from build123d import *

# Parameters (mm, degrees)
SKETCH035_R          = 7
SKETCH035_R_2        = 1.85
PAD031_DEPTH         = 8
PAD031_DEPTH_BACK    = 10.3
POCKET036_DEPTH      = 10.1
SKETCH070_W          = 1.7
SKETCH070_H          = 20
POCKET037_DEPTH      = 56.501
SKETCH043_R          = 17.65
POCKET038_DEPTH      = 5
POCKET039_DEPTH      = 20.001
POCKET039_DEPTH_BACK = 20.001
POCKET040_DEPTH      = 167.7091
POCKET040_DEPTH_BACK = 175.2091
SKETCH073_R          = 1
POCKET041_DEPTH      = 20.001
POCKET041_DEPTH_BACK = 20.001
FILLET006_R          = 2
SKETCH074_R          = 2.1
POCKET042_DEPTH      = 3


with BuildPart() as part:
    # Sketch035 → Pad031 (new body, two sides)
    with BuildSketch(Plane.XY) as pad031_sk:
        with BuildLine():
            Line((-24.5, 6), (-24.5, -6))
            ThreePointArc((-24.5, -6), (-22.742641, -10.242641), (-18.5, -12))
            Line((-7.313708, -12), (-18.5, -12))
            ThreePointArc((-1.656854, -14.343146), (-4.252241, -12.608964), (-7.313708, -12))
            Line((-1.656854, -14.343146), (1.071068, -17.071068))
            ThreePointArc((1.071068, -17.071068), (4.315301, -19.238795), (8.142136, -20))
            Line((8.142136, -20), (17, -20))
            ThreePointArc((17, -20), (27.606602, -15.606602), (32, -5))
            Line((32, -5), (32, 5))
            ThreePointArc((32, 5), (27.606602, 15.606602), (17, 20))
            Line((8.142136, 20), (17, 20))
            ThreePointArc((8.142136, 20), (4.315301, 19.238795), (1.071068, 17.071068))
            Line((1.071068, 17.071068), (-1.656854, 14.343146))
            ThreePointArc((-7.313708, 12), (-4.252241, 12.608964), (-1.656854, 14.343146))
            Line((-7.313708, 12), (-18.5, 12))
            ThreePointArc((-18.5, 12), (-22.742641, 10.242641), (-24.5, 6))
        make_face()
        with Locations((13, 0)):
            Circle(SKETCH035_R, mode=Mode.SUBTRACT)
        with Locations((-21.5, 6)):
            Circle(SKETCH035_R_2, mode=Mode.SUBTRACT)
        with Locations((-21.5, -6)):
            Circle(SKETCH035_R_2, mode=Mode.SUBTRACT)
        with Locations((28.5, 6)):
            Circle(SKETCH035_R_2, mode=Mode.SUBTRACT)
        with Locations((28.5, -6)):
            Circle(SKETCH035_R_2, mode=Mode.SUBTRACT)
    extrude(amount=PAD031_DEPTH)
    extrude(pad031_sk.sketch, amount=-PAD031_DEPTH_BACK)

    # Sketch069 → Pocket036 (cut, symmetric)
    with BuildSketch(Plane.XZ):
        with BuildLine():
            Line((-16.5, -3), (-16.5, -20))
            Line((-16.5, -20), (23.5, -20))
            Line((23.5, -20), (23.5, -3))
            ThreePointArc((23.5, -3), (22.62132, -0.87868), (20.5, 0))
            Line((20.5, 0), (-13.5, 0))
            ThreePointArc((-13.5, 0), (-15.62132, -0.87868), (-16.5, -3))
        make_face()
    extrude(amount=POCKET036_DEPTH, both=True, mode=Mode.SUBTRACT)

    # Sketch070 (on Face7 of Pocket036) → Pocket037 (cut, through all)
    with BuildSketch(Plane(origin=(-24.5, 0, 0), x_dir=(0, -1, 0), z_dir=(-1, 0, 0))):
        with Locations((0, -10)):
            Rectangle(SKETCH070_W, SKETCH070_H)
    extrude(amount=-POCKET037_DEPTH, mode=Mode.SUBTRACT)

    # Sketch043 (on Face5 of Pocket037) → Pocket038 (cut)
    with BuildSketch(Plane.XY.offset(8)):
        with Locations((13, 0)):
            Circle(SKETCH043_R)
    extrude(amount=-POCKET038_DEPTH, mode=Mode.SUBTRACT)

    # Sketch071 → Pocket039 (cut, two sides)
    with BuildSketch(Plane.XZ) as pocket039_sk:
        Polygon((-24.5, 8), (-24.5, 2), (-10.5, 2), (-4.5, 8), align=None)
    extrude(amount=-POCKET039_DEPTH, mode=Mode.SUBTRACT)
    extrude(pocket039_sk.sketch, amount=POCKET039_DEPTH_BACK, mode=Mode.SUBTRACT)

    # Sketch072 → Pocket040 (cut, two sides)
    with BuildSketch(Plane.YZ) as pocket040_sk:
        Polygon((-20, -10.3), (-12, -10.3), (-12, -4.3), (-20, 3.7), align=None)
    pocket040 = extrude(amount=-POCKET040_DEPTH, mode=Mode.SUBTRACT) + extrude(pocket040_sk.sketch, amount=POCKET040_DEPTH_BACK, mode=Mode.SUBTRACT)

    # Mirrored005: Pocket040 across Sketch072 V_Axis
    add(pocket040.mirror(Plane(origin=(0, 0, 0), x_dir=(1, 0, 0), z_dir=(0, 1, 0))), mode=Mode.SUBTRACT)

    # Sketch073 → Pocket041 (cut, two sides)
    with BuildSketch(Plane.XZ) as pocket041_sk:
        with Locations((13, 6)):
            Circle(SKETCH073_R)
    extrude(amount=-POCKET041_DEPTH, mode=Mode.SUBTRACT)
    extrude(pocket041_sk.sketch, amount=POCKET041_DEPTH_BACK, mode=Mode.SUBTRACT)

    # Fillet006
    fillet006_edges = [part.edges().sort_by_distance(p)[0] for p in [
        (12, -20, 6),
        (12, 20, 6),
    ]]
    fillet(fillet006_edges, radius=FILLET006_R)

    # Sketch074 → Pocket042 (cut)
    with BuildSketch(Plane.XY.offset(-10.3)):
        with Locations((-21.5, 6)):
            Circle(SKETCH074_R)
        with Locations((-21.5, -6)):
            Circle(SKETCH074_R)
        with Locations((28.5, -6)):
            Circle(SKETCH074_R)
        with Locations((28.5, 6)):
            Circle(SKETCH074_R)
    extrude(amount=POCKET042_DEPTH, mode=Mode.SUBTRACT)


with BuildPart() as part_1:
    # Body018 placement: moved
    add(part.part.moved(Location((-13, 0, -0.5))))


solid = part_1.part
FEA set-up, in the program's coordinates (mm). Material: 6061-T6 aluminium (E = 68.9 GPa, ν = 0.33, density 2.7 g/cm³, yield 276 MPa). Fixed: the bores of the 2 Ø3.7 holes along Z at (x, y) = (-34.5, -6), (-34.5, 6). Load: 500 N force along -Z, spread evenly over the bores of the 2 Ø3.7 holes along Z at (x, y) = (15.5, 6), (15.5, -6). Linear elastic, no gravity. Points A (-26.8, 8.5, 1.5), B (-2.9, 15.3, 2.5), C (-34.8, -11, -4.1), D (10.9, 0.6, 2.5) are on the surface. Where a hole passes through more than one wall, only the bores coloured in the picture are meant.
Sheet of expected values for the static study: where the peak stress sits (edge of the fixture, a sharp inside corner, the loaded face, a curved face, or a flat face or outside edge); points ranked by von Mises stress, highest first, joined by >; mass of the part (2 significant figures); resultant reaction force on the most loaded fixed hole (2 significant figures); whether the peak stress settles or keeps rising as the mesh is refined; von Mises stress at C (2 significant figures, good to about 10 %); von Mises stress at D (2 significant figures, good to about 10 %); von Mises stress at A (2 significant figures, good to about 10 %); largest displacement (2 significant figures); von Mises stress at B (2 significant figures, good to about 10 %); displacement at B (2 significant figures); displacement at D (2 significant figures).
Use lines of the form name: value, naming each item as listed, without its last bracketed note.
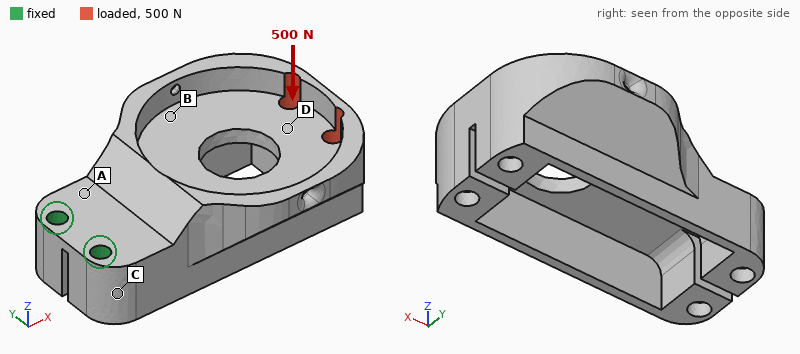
where the peak stress sits: edge of the fixture
points ranked by von Mises stress, highest first, joined by >: A > C > D > B
mass of the part: 30 g
resultant reaction force on the most loaded fixed hole: 370 N
whether the peak stress settles or keeps rising as the mesh is refined: keeps rising
von Mises stress at C: 42 MPa
von Mises stress at D: 30 MPa
von Mises stress at A: 85 MPa
largest displacement: 0.32 mm
von Mises stress at B: 13 MPa
displacement at B: 0.14 mm
displacement at D: 0.25 mm
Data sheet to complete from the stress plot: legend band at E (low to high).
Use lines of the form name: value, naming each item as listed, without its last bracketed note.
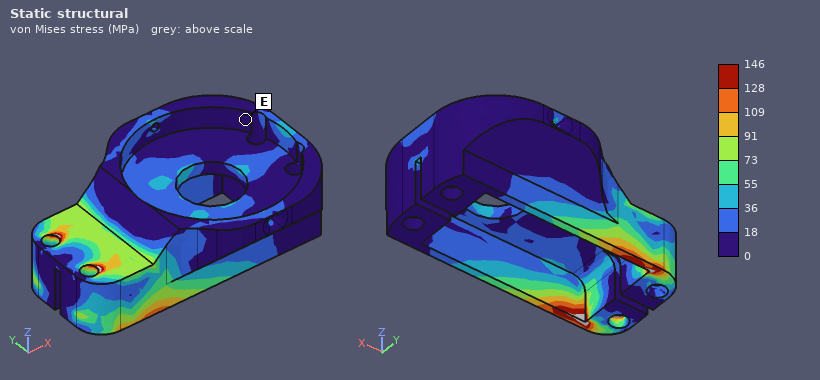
legend band at E: 0 to 18 MPa
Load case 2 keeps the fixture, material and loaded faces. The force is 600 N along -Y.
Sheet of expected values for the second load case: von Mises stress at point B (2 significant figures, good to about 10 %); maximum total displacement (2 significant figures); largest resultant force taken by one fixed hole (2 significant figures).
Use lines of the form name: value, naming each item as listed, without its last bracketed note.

von Mises stress at point B: 9.4 MPa
maximum total displacement: 0.15 mm
largest resultant force taken by one fixed hole: 1.7 kN
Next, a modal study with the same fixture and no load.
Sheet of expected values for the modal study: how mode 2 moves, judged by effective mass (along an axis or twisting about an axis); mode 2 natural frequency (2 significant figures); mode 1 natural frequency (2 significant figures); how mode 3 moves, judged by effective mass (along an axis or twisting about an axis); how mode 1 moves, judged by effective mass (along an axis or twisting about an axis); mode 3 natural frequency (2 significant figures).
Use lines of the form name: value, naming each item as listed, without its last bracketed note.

how mode 2 moves, judged by effective mass: along Y
mode 2 natural frequency: 2800 Hz
mode 1 natural frequency: 1900 Hz
how mode 3 moves, judged by effective mass: along Y
how mode 1 moves, judged by effective mass: along Z
mode 3 natural frequency: 4700 Hz
